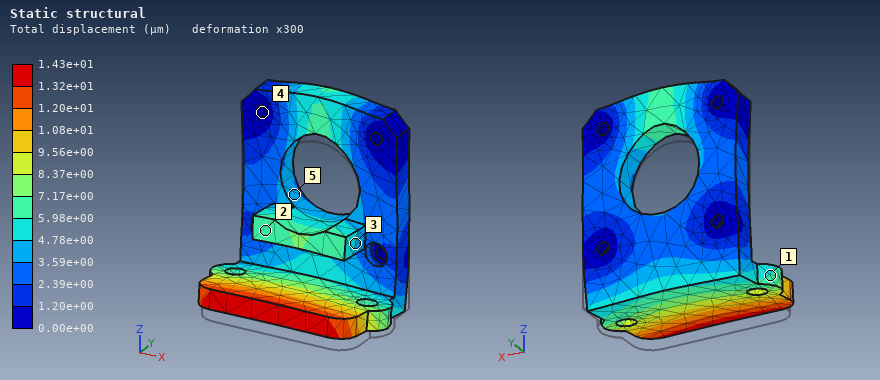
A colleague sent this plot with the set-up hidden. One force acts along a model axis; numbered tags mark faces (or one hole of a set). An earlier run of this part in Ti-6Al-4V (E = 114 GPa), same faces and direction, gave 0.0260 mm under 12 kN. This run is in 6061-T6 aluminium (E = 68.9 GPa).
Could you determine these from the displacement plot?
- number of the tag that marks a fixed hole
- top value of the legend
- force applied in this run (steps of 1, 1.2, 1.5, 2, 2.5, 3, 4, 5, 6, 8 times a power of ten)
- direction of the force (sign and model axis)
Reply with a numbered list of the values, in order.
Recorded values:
1. 4
2. 1.43e+01 µm
3. 4 kN
4. +Z
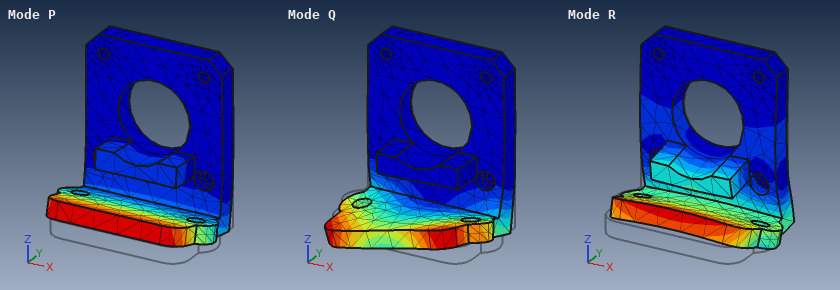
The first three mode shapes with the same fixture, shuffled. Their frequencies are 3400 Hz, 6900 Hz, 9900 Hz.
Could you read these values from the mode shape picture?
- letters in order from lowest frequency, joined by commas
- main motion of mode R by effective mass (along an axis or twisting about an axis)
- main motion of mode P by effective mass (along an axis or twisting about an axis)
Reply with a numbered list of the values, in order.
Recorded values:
1. P, Q, R
2. along Y
3. along Z
